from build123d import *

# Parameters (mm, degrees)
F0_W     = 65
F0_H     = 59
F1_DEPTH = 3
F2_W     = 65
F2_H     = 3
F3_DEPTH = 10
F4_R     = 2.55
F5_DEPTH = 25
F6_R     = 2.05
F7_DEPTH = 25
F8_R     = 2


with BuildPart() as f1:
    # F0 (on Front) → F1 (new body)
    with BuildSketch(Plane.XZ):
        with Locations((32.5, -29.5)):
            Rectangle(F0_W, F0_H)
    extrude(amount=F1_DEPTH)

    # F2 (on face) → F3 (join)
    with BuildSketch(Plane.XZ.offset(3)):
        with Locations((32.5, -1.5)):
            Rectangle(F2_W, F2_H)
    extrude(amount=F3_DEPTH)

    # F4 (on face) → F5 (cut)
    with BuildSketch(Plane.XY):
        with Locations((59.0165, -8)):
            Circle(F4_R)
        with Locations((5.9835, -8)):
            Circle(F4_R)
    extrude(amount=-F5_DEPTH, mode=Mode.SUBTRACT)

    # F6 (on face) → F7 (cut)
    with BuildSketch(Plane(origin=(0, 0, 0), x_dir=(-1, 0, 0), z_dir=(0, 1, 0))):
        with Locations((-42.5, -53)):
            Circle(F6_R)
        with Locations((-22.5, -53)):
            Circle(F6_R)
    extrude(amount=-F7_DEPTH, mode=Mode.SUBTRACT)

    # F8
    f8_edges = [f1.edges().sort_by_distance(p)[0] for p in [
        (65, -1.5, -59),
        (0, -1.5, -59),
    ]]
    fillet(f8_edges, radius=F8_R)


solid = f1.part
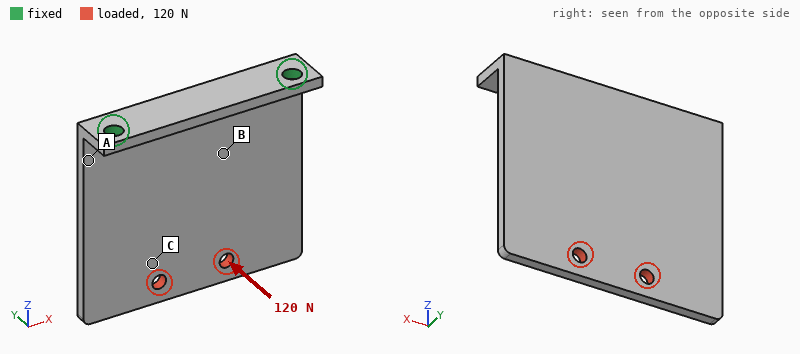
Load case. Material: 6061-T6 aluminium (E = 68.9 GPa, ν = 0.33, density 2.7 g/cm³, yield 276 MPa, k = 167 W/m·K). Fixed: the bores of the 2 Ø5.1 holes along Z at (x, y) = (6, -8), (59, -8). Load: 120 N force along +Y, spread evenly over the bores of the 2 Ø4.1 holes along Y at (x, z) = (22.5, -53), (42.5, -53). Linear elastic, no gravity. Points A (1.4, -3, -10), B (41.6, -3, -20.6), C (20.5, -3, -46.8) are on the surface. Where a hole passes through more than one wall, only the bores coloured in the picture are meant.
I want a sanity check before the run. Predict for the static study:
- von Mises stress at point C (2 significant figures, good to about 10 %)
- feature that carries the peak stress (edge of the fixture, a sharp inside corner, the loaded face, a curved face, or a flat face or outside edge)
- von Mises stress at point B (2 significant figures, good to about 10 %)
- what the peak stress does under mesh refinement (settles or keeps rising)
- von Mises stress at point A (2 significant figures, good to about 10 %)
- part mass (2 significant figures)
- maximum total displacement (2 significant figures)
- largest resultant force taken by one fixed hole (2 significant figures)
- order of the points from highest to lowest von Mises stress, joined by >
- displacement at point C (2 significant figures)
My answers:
17 MPa
edge of the fixture
38 MPa
keeps rising
56 MPa
36 g
0.95 mm
63 N
A > B > C
0.68 mm
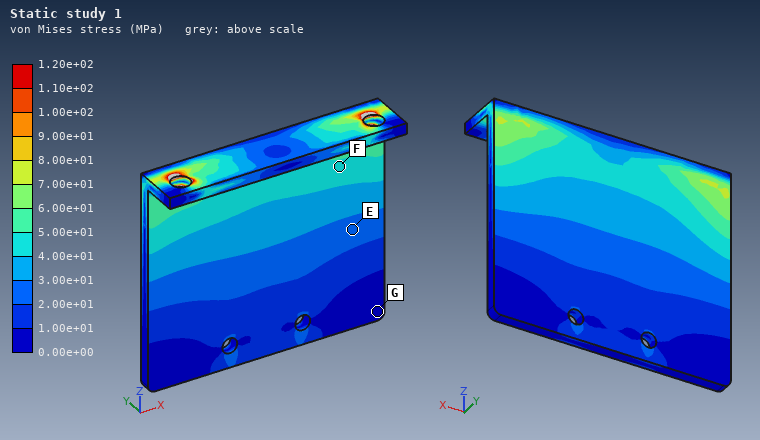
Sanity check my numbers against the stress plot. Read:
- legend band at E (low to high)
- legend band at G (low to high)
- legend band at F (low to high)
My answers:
2.00e+01 to 3.00e+01 MPa
0.00e+00 to 1.00e+01 MPa
4.00e+01 to 5.00e+01 MPa
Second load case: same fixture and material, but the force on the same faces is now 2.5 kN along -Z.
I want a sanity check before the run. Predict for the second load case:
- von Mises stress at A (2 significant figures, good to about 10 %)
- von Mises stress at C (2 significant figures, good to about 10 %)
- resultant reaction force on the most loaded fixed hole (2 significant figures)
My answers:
32 MPa
26 MPa
1.3 kN
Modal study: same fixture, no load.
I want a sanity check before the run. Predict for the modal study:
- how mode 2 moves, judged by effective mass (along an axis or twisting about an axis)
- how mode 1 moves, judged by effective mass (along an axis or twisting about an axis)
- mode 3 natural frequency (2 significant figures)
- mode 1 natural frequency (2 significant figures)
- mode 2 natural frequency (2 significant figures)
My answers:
twisting about Z
along Y
3900 Hz
600 Hz
1600 Hz
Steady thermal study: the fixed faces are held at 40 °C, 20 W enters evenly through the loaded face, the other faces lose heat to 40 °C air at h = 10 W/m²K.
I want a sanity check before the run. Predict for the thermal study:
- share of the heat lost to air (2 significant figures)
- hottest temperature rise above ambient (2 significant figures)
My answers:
9.9 %
43 K
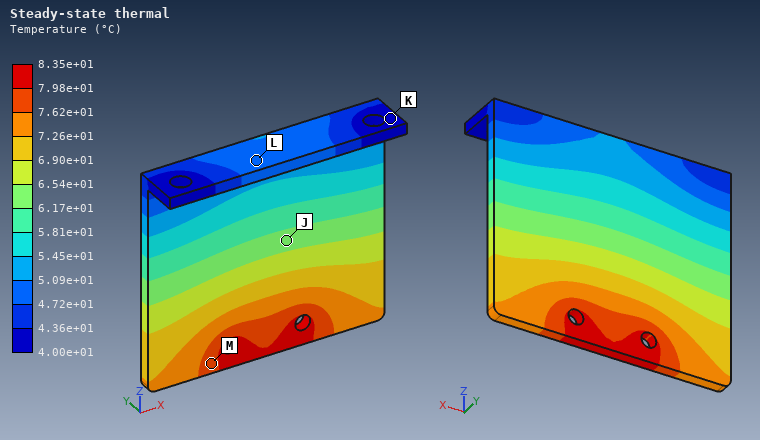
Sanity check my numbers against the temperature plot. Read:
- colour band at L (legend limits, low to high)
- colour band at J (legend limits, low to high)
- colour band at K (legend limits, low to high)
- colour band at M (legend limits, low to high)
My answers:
4.72e+01 to 5.09e+01 °C
6.17e+01 to 6.54e+01 °C
4.00e+01 to 4.36e+01 °C
7.62e+01 to 7.98e+01 °C
